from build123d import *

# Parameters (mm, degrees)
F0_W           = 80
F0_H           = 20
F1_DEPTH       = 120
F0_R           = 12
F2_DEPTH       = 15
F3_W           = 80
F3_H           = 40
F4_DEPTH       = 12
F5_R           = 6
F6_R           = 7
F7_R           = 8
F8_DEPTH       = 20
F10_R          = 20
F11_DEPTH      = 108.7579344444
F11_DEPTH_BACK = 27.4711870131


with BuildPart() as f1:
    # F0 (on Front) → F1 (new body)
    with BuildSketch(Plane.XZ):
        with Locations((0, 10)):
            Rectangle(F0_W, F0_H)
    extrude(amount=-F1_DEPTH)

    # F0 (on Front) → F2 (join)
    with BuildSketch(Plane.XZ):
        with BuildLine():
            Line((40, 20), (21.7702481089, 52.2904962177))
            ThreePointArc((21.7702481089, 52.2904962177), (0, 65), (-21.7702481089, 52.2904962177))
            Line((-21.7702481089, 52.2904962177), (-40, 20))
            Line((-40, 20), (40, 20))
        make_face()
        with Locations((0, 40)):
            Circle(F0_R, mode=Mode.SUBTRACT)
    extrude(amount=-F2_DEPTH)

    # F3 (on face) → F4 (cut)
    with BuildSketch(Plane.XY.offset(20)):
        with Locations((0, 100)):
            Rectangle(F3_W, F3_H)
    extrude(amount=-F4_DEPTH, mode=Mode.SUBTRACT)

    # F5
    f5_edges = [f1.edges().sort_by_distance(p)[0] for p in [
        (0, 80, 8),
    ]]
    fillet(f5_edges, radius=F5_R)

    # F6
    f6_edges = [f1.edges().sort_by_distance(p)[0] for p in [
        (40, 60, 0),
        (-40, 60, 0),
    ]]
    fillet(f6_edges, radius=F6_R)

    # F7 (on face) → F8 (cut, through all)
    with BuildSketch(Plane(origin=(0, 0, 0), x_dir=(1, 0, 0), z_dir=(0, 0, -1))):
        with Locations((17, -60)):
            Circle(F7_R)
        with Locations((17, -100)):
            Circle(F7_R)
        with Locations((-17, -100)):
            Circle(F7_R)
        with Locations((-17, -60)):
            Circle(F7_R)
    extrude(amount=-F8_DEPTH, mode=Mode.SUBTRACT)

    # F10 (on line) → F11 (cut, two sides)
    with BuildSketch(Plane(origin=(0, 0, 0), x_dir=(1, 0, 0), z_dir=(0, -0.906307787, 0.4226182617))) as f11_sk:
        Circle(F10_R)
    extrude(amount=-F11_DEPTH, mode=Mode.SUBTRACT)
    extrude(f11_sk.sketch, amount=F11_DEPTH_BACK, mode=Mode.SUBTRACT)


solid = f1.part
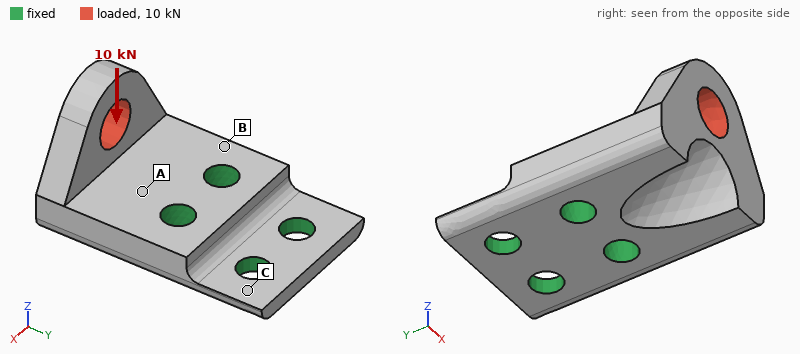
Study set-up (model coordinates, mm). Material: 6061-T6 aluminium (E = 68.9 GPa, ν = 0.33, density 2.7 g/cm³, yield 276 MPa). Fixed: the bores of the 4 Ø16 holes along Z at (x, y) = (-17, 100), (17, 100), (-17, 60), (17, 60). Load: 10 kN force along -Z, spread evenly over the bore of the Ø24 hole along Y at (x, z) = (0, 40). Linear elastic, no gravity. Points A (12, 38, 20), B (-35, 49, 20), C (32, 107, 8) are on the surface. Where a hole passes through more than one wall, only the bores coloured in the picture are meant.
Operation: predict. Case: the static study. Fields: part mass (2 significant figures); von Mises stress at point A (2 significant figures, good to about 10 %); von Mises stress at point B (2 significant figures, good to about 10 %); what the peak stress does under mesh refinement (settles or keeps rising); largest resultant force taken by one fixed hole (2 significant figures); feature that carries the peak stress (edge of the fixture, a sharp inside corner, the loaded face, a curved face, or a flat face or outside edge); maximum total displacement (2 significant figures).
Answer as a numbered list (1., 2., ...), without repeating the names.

1. 420 g
2. 62 MPa
3. 52 MPa
4. keeps rising
5. 5.4 kN
6. edge of the fixture
7. 0.28 mm
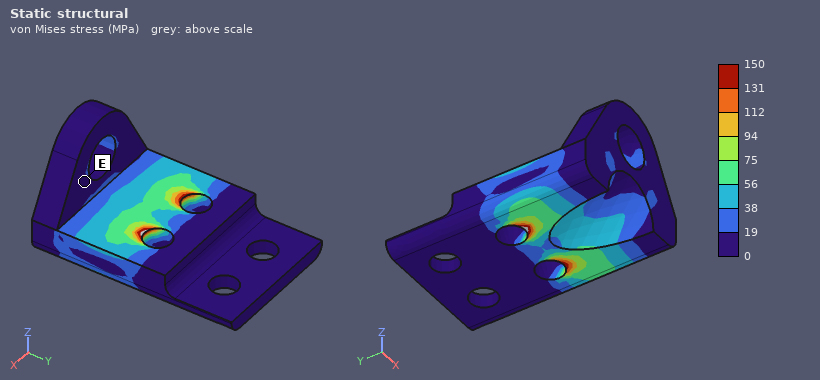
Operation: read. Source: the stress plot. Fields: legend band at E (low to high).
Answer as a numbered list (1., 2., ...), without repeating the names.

1. 0 to 19 MPa
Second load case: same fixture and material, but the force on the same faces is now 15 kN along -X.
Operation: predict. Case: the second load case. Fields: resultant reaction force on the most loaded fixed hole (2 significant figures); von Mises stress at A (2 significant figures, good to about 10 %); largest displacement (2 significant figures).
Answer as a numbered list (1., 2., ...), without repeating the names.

1. 18 kN
2. 75 MPa
3. 0.24 mm
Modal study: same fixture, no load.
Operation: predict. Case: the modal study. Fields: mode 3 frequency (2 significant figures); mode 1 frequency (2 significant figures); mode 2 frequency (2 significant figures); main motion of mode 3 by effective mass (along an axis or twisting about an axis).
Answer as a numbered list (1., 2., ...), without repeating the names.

1. 6000 Hz
2. 2800 Hz
3. 4300 Hz
4. along Z
